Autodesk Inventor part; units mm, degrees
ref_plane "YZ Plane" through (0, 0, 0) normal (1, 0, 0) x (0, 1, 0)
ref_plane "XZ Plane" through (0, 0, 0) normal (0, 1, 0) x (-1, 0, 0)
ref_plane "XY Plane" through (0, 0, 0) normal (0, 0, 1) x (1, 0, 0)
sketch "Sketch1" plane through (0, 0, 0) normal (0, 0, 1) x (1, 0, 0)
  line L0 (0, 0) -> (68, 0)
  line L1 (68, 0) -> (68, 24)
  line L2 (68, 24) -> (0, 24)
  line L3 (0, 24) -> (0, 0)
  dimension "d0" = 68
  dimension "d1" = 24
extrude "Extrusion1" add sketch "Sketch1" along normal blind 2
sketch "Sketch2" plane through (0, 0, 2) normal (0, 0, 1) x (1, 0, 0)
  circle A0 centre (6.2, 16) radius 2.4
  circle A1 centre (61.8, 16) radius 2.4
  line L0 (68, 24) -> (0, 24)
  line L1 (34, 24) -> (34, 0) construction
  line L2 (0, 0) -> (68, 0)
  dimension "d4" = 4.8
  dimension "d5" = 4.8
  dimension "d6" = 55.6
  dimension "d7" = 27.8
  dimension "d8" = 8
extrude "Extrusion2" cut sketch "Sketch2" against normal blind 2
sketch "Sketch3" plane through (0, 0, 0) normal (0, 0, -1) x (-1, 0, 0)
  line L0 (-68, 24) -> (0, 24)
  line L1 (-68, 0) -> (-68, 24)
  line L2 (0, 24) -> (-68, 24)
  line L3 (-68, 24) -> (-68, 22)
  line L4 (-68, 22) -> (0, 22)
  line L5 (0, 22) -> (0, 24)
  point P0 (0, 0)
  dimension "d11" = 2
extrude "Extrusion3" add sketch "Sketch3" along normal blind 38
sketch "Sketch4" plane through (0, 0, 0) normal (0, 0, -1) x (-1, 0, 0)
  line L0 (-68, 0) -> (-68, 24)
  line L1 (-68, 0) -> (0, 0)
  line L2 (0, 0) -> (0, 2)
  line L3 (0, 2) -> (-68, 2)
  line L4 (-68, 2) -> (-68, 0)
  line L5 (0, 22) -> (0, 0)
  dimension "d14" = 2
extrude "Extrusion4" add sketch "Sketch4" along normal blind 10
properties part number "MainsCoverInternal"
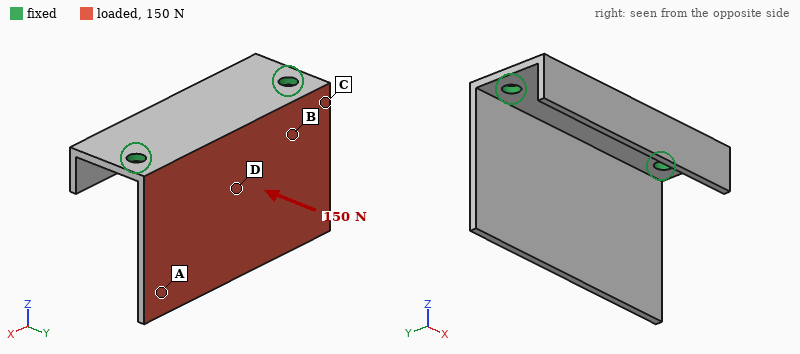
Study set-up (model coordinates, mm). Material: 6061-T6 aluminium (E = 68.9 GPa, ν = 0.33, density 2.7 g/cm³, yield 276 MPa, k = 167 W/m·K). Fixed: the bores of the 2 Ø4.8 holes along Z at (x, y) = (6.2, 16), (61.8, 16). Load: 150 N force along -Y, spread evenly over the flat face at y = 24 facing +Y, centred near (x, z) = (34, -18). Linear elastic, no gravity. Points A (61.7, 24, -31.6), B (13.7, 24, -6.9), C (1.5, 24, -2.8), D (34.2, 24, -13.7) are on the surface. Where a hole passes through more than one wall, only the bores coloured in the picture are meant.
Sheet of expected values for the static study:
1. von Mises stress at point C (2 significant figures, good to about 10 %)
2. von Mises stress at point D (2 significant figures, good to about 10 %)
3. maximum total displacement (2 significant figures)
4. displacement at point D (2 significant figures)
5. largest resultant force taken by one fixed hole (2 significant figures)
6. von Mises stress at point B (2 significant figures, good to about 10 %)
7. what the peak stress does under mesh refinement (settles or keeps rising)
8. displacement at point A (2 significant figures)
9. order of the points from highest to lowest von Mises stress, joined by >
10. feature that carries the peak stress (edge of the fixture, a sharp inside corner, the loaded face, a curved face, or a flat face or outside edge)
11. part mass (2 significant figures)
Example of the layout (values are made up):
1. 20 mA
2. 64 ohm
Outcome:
1. 52 MPa
2. 21 MPa
3. 0.56 mm
4. 0.17 mm
5. 75 N
6. 36 MPa
7. keeps rising
8. 0.44 mm
9. C > B > D > A
10. edge of the fixture
11. 26 g
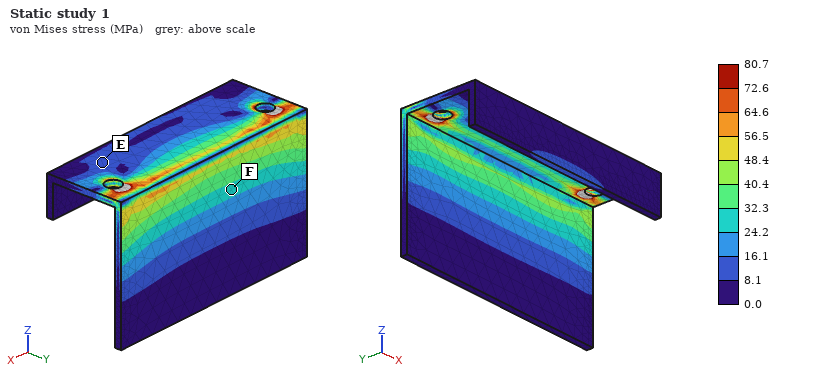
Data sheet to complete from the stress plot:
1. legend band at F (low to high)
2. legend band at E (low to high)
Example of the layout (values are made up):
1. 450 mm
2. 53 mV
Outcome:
1. 24.2 to 32.3 MPa
2. 8.1 to 16.1 MPa
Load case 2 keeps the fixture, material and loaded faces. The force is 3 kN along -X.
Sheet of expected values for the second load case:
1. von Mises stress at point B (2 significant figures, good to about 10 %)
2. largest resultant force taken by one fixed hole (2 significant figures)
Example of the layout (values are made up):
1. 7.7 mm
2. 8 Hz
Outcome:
1. 37 MPa
2. 1.9 kN
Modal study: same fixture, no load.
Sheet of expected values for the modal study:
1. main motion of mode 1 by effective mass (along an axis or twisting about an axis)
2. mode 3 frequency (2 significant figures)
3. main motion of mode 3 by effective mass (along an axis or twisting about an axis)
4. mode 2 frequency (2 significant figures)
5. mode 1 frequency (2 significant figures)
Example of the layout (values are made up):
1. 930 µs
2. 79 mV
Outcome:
1. along Y
2. 2800 Hz
3. along Z
4. 1600 Hz
5. 840 Hz
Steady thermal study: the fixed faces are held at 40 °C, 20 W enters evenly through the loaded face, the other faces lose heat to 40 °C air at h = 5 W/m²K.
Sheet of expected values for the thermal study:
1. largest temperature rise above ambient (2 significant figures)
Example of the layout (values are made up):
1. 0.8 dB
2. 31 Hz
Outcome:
1. 28 K
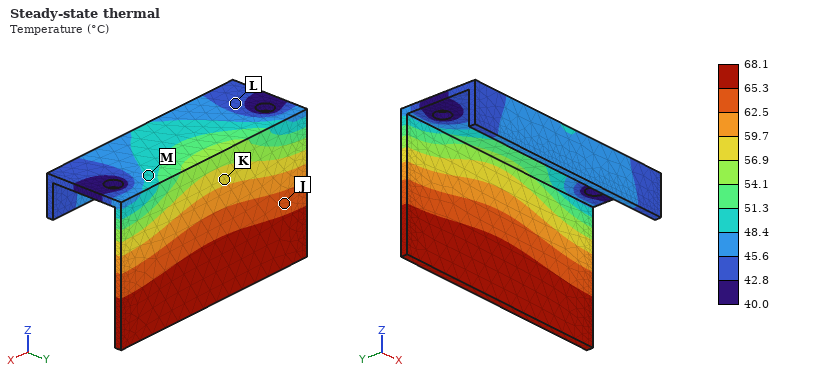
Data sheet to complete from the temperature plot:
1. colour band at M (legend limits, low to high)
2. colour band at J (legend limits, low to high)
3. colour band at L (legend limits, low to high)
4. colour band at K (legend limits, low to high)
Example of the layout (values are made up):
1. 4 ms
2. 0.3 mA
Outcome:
1. 48.4 to 51.3 °C
2. 62.5 to 65.3 °C
3. 42.8 to 45.6 °C
4. 56.9 to 59.7 °C
